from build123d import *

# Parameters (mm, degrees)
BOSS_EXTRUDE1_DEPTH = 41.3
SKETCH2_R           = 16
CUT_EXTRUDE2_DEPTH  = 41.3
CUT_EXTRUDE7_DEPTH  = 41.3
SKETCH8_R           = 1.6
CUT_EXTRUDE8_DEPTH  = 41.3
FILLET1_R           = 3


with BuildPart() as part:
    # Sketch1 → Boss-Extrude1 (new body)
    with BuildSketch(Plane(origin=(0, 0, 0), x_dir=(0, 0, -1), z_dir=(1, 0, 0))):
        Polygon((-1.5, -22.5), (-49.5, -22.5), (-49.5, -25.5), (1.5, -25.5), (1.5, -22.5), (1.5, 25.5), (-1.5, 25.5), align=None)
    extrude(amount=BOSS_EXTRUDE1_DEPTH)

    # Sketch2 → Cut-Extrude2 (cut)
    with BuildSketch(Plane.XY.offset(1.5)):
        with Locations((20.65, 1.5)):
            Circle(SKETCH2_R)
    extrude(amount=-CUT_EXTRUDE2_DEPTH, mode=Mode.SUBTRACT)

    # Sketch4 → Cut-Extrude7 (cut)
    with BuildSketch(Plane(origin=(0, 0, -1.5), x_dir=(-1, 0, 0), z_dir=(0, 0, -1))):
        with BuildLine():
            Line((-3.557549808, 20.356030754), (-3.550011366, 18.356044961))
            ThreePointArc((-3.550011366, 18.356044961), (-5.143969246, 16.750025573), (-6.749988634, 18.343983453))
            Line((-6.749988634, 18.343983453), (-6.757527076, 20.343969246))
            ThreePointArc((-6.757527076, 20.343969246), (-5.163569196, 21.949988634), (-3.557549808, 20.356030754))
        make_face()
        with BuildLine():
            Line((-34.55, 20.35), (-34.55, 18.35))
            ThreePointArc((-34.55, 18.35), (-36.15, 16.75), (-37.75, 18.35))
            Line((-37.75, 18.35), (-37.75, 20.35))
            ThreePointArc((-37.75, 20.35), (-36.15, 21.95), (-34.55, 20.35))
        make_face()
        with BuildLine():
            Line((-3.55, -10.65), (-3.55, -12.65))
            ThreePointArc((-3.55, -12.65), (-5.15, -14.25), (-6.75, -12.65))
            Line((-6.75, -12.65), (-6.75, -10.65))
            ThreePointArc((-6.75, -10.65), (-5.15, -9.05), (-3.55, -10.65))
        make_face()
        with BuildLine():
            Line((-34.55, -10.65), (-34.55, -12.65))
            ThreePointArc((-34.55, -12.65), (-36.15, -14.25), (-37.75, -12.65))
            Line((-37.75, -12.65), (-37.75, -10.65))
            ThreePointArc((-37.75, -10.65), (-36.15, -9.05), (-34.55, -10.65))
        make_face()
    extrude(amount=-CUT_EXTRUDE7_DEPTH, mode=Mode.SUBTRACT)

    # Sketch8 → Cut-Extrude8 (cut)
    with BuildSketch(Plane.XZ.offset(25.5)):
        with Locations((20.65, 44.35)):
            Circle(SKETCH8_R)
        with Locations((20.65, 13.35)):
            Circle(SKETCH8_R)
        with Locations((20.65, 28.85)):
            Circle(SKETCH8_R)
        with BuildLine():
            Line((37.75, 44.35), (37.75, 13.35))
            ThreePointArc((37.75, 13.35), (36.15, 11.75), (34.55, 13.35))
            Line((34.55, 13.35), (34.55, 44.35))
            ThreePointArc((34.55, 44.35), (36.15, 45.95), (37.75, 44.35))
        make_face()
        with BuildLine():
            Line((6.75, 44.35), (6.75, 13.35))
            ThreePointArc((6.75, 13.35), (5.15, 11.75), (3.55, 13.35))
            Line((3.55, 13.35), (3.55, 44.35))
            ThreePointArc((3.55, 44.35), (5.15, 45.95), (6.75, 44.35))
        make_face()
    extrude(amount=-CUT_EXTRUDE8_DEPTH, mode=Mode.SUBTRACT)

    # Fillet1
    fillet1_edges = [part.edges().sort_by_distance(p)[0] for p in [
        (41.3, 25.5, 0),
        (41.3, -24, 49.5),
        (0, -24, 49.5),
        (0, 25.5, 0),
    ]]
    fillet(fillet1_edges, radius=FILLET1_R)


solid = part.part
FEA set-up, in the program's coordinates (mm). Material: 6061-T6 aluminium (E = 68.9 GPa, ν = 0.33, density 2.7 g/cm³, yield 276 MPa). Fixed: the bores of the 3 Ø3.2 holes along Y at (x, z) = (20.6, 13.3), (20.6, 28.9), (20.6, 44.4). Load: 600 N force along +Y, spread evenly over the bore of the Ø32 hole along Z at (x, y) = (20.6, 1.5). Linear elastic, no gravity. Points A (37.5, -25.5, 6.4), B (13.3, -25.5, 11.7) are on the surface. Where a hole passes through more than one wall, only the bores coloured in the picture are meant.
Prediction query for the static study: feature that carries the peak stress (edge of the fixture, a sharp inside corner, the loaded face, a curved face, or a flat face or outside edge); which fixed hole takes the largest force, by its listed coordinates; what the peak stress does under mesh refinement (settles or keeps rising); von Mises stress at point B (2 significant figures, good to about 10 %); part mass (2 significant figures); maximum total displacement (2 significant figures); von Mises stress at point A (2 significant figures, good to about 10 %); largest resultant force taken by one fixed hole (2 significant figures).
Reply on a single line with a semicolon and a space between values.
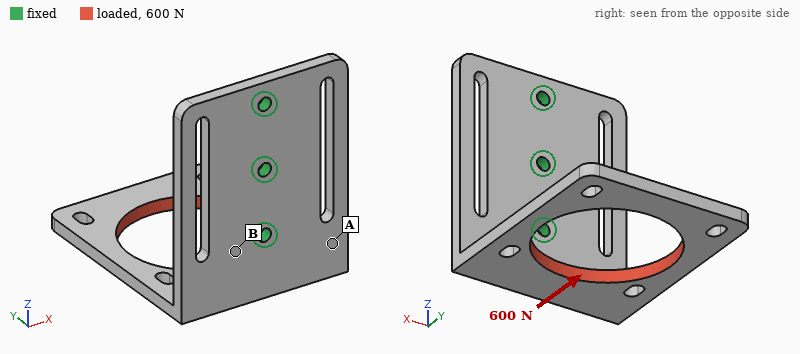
edge of the fixture; (20.6, 13.3); keeps rising; 90 MPa; 24 g; 0.56 mm; 36 MPa; 810 N
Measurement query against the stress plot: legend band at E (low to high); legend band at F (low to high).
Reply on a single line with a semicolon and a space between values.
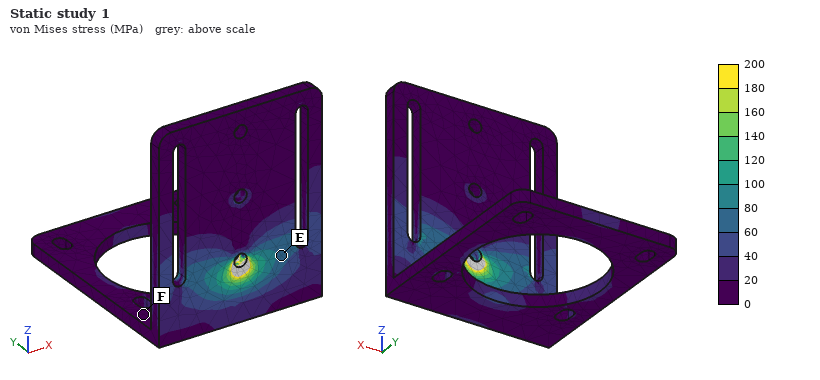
60 to 80 MPa; 0 to 20 MPa
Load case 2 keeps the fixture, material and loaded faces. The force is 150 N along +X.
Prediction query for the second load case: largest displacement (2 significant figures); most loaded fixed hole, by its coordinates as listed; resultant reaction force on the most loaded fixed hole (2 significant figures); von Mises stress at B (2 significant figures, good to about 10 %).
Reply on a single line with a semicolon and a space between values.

0.36 mm; (20.6, 13.3); 210 N; 39 MPa
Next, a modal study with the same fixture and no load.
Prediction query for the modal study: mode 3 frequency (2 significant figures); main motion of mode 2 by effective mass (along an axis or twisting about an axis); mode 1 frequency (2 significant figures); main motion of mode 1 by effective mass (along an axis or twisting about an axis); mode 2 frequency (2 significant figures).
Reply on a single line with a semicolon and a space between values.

2000 Hz; along X; 660 Hz; along Z; 1200 Hz
